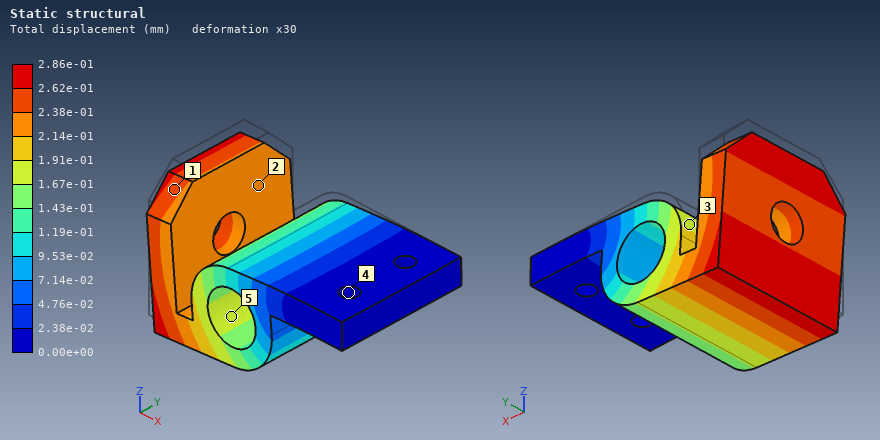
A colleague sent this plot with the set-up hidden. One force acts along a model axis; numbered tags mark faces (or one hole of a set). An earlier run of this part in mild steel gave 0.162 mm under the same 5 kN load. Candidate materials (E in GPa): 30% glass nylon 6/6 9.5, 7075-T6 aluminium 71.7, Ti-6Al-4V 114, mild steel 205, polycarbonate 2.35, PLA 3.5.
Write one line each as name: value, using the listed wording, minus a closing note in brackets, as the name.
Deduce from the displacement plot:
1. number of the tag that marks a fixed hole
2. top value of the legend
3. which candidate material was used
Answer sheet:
number of the tag that marks a fixed hole: 4
top value of the legend: 2.86e-01 mm
which candidate material was used: Ti-6Al-4V
